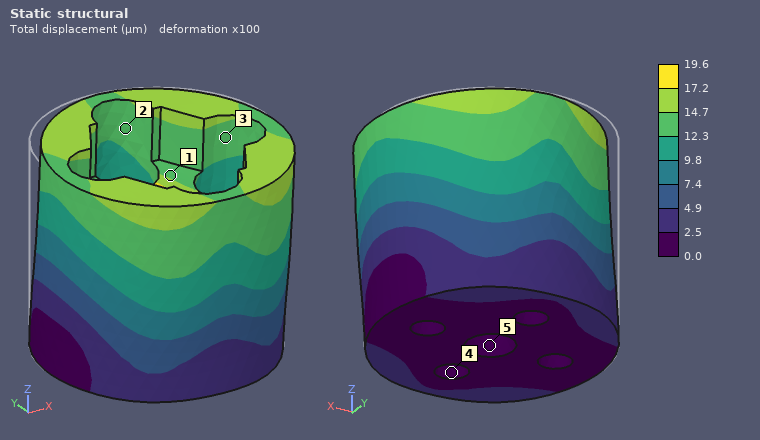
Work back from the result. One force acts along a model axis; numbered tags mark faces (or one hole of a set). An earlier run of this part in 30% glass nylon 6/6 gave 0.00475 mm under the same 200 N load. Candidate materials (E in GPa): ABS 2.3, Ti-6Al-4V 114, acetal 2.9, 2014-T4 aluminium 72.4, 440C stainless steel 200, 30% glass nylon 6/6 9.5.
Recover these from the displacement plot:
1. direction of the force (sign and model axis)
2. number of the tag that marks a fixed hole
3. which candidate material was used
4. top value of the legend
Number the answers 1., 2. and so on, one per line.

1. -Y
2. 4
3. ABS
4. 19.6 µm
